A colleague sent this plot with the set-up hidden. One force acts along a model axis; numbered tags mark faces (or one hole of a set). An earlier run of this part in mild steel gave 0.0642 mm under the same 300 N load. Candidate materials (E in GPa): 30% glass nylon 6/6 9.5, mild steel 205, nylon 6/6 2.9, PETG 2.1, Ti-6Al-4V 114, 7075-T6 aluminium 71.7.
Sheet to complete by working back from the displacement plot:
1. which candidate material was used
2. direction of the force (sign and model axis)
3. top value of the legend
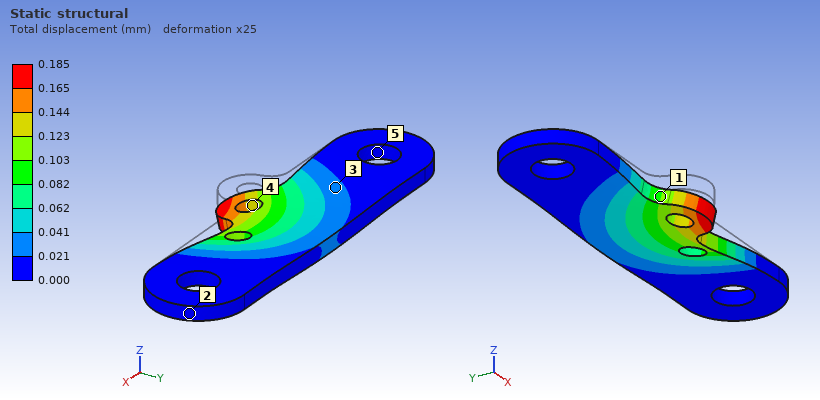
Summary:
7075-T6 aluminium
-Z
0.185 mm
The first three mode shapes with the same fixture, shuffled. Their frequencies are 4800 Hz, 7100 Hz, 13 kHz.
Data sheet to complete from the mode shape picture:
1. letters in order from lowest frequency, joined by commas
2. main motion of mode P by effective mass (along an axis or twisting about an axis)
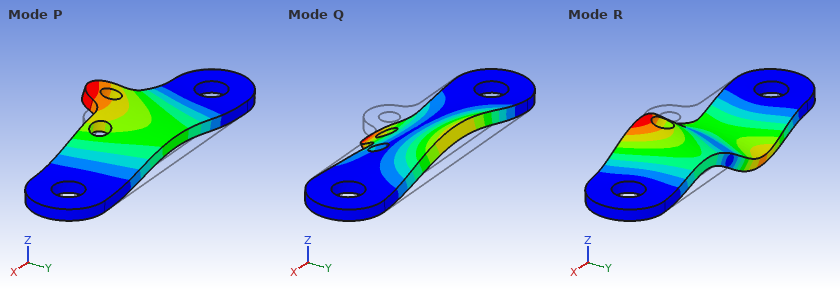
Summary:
P, Q, R
along Z
